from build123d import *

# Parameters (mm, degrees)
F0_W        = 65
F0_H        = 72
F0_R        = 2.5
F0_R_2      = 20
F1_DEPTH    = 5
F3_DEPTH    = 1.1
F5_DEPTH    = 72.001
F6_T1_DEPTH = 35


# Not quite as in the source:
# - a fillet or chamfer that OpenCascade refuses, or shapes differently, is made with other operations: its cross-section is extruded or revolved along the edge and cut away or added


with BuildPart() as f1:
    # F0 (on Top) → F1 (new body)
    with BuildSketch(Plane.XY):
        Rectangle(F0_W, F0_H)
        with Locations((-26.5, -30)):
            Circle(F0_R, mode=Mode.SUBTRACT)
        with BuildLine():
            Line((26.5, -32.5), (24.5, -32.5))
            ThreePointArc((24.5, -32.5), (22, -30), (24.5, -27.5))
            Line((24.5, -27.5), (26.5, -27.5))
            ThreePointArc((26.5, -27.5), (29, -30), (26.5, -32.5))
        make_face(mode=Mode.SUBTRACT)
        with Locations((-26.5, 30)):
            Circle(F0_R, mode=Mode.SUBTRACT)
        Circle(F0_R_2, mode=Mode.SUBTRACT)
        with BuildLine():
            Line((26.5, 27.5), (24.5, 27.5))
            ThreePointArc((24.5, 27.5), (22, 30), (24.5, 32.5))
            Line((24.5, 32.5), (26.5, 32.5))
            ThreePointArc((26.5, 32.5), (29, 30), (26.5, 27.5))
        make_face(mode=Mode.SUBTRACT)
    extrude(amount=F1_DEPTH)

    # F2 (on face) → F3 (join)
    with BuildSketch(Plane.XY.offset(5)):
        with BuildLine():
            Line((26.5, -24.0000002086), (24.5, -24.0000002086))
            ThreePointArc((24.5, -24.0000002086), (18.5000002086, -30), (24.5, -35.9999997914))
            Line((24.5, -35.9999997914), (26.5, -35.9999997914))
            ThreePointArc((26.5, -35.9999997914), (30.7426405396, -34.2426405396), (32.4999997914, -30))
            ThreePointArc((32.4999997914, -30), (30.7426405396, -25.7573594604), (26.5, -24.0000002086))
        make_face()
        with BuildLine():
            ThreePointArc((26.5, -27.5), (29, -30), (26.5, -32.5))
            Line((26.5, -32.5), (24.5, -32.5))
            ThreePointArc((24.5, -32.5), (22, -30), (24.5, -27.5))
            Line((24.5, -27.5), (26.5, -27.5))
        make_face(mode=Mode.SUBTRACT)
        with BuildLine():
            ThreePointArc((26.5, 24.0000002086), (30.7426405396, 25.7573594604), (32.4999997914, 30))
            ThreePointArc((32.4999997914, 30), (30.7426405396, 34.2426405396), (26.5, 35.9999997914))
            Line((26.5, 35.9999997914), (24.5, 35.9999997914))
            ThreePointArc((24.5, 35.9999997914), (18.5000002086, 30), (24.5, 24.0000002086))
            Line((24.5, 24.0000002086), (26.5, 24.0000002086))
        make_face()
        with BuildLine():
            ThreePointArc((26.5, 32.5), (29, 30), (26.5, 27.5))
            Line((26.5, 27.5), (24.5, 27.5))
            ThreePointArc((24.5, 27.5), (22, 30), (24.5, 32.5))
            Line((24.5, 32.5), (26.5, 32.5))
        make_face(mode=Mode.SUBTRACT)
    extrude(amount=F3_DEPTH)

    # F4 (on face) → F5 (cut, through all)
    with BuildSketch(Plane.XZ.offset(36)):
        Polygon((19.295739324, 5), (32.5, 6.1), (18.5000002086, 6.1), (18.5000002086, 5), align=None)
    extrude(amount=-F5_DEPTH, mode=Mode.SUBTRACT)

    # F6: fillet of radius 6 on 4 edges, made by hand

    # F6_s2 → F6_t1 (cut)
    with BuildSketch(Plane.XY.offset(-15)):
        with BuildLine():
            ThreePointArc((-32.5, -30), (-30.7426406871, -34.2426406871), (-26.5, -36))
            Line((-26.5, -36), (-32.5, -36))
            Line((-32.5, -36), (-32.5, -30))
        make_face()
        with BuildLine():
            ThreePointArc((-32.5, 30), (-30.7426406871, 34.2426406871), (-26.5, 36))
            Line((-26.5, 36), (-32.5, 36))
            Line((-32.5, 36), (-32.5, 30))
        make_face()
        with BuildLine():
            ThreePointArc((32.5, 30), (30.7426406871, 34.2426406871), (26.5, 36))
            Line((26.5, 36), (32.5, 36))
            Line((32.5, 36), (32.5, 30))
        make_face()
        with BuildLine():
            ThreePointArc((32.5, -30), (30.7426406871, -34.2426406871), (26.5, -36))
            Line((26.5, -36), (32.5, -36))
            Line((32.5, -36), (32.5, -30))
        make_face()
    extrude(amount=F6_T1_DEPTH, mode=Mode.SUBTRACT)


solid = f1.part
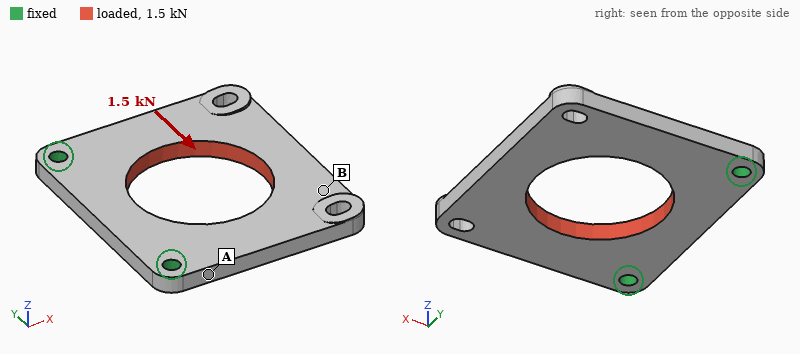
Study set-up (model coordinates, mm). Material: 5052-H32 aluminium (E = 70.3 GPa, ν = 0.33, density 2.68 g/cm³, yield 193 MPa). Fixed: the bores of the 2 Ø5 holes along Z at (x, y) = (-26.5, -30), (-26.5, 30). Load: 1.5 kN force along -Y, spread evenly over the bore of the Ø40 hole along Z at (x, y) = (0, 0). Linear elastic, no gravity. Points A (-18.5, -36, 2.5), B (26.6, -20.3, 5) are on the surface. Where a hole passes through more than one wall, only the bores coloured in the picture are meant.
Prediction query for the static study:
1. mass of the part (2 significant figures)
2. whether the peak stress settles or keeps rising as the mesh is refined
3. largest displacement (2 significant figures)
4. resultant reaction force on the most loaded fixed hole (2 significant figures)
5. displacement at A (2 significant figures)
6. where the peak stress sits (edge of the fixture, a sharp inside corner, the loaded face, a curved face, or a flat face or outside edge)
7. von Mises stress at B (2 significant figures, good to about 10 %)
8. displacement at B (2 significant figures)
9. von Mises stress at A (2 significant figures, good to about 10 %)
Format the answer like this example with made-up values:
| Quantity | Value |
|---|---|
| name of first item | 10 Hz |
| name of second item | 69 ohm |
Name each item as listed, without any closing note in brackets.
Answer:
| Quantity | Value |
|---|---|
| mass of the part | 44 g |
| whether the peak stress settles or keeps rising as the mesh is refined | keeps rising |
| largest displacement | 33 µm |
| resultant reaction force on the most loaded fixed hole | 940 N |
| displacement at A | 5.6 µm |
| where the peak stress sits | edge of the fixture |
| von Mises stress at B | 5.5 MPa |
| displacement at B | 31 µm |
| von Mises stress at A | 19 MPa |
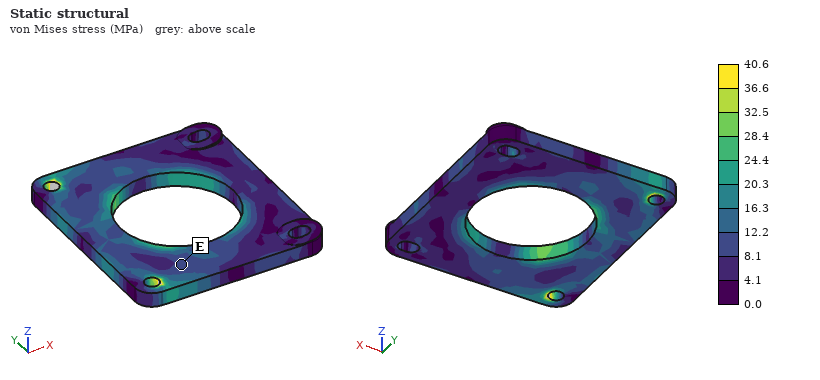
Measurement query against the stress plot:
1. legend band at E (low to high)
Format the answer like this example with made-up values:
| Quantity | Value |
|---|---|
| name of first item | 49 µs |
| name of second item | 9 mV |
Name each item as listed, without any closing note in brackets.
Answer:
| Quantity | Value |
|---|---|
| legend band at E | 8.1 to 12.2 MPa |
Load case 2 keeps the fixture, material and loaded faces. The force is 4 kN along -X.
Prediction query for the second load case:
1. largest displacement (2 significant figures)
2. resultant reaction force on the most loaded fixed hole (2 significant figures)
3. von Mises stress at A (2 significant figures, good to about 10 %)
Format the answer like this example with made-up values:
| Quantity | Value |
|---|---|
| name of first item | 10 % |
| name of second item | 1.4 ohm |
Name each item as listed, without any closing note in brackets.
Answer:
| Quantity | Value |
|---|---|
| largest displacement | 18 µm |
| resultant reaction force on the most loaded fixed hole | 2.0 kN |
| von Mises stress at A | 22 MPa |
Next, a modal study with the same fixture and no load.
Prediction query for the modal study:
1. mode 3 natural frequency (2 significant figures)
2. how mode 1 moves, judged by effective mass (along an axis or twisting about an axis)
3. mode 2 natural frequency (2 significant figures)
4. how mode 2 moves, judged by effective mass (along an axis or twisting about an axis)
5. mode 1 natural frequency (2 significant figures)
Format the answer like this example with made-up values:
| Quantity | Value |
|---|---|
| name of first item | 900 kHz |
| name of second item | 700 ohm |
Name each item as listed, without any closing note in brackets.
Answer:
| Quantity | Value |
|---|---|
| mode 3 natural frequency | 5600 Hz |
| how mode 1 moves, judged by effective mass | along Z |
| mode 2 natural frequency | 2200 Hz |
| how mode 2 moves, judged by effective mass | twisting about X |
| mode 1 natural frequency | 950 Hz |
